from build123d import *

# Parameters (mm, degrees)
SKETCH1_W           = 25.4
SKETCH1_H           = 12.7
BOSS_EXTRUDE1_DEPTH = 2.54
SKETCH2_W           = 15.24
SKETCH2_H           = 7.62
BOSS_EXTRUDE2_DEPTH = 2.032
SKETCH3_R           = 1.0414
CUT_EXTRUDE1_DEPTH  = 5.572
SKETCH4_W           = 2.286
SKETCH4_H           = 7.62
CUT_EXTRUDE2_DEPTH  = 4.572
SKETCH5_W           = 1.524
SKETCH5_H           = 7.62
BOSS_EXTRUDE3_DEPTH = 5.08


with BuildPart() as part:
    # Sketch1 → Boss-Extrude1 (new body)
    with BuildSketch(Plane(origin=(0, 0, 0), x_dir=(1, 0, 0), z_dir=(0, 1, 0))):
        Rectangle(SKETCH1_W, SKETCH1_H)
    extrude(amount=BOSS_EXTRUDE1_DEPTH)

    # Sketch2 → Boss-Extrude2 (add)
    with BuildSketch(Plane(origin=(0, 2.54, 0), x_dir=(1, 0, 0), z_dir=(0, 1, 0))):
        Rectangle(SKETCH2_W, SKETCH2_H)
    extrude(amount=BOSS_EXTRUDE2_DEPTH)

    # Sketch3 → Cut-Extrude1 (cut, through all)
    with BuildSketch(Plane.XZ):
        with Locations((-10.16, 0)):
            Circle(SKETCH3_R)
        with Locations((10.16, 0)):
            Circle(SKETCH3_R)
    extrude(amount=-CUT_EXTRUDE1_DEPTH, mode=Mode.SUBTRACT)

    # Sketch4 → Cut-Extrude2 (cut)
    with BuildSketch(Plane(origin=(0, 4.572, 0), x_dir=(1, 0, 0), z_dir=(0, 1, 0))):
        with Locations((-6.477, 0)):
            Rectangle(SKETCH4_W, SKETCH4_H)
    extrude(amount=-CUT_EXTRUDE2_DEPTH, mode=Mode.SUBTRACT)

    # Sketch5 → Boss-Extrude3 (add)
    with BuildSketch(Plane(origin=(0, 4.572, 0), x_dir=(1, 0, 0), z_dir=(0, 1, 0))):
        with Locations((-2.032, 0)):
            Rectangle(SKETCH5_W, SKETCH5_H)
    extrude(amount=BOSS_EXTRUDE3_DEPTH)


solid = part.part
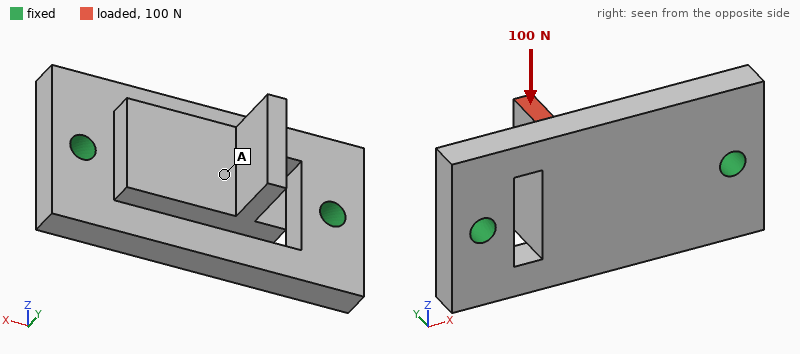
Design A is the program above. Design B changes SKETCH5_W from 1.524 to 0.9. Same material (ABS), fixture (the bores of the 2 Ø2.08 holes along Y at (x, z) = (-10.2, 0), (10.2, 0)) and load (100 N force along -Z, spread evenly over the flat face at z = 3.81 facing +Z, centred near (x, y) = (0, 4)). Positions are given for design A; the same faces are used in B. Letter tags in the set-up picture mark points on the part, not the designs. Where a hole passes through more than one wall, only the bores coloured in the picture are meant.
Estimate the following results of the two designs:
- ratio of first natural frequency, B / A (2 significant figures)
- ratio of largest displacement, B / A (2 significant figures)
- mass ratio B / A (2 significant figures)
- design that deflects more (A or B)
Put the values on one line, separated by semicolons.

1.0; 0.92; 0.98; A
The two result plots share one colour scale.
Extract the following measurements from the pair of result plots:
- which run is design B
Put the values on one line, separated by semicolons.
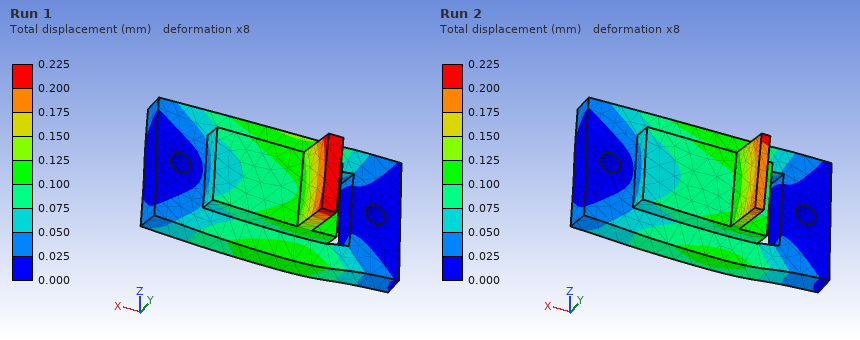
Run 2
